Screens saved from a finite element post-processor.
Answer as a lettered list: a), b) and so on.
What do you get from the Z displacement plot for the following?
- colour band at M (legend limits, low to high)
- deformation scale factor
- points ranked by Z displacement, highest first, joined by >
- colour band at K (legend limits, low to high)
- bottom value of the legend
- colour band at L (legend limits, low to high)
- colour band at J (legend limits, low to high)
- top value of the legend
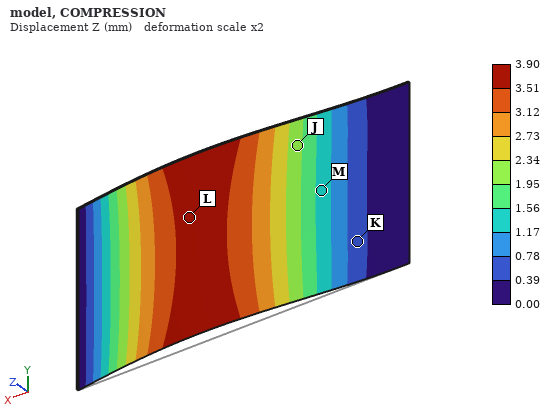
a) 1.17 to 1.56 mm
b) 2
c) L > J > M > K
d) 0.39 to 0.78 mm
e) 0.00 mm
f) 3.51 to 3.90 mm
g) 1.95 to 2.34 mm
h) 3.90 mm
